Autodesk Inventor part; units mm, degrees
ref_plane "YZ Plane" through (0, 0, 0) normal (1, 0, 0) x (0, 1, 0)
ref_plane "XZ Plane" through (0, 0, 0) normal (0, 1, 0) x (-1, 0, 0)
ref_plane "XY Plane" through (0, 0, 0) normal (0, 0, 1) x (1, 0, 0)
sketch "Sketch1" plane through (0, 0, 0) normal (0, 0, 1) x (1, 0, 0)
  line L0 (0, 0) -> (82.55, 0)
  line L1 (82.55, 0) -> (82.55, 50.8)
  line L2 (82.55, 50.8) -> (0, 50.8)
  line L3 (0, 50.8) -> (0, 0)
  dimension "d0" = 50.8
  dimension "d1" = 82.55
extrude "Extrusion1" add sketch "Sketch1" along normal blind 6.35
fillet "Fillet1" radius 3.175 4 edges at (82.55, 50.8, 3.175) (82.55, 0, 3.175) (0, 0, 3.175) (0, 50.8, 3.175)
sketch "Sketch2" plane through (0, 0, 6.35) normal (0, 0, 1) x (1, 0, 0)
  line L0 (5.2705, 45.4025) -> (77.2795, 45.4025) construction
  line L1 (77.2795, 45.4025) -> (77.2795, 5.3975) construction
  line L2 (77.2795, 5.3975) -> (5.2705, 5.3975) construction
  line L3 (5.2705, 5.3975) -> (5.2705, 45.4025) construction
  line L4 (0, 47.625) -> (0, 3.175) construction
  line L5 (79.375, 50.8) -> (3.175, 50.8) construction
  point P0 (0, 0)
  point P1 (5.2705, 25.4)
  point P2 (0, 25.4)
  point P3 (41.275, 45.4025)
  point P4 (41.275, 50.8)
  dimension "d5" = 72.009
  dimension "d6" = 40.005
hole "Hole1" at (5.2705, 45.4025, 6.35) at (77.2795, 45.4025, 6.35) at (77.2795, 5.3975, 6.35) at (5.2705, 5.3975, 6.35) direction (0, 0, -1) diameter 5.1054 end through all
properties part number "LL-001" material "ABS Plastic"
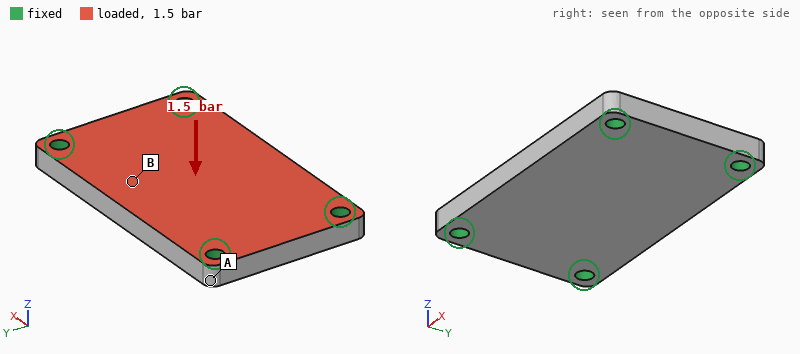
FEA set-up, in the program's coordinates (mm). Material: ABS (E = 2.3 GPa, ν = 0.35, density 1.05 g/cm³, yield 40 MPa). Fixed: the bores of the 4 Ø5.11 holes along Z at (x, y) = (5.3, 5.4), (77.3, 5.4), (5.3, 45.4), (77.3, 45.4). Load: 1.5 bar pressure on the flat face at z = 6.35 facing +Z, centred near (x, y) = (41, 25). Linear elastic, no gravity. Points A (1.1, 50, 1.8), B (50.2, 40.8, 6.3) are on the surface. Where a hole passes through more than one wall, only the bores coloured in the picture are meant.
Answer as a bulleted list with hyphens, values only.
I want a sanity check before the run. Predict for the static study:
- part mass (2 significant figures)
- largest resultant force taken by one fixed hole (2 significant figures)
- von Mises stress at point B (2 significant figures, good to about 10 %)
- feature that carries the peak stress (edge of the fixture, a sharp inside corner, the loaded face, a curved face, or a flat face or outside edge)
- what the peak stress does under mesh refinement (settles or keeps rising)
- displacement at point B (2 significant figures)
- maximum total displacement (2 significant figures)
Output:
- 27 g
- 150 N
- 4.3 MPa
- edge of the fixture
- keeps rising
- 0.25 mm
- 0.28 mm
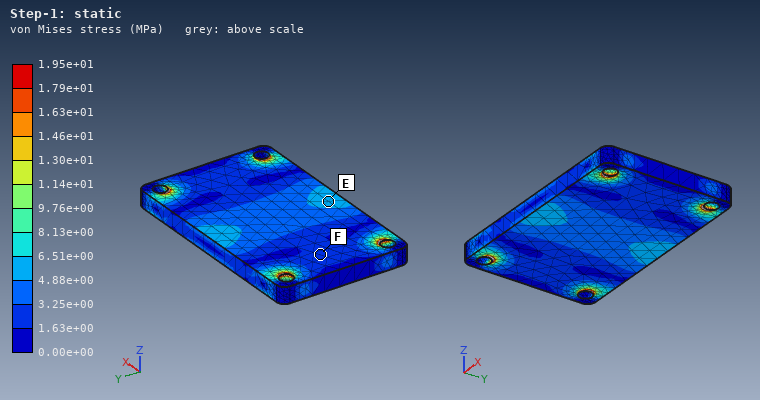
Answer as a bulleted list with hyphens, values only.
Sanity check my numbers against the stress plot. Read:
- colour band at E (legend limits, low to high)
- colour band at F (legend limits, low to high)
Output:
- 4.88e+00 to 6.51e+00 MPa
- 1.63e+00 to 3.25e+00 MPa
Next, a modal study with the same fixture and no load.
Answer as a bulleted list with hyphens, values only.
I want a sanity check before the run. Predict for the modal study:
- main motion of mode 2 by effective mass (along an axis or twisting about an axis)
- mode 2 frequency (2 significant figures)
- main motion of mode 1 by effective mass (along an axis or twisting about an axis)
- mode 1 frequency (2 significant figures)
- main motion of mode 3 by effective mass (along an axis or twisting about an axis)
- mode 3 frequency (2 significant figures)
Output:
- twisting about X
- 2500 Hz
- along Z
- 1600 Hz
- twisting about Y
- 4100 Hz
